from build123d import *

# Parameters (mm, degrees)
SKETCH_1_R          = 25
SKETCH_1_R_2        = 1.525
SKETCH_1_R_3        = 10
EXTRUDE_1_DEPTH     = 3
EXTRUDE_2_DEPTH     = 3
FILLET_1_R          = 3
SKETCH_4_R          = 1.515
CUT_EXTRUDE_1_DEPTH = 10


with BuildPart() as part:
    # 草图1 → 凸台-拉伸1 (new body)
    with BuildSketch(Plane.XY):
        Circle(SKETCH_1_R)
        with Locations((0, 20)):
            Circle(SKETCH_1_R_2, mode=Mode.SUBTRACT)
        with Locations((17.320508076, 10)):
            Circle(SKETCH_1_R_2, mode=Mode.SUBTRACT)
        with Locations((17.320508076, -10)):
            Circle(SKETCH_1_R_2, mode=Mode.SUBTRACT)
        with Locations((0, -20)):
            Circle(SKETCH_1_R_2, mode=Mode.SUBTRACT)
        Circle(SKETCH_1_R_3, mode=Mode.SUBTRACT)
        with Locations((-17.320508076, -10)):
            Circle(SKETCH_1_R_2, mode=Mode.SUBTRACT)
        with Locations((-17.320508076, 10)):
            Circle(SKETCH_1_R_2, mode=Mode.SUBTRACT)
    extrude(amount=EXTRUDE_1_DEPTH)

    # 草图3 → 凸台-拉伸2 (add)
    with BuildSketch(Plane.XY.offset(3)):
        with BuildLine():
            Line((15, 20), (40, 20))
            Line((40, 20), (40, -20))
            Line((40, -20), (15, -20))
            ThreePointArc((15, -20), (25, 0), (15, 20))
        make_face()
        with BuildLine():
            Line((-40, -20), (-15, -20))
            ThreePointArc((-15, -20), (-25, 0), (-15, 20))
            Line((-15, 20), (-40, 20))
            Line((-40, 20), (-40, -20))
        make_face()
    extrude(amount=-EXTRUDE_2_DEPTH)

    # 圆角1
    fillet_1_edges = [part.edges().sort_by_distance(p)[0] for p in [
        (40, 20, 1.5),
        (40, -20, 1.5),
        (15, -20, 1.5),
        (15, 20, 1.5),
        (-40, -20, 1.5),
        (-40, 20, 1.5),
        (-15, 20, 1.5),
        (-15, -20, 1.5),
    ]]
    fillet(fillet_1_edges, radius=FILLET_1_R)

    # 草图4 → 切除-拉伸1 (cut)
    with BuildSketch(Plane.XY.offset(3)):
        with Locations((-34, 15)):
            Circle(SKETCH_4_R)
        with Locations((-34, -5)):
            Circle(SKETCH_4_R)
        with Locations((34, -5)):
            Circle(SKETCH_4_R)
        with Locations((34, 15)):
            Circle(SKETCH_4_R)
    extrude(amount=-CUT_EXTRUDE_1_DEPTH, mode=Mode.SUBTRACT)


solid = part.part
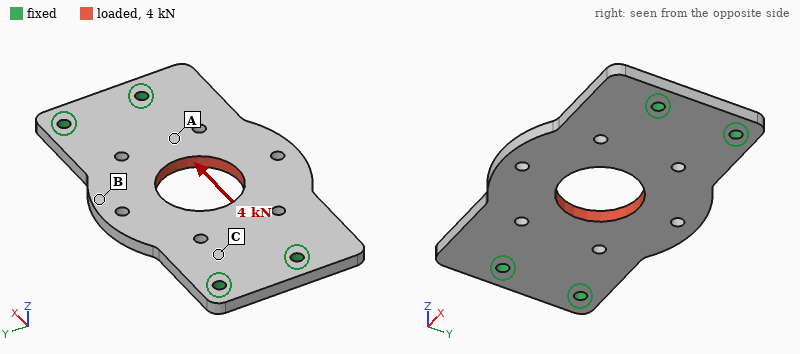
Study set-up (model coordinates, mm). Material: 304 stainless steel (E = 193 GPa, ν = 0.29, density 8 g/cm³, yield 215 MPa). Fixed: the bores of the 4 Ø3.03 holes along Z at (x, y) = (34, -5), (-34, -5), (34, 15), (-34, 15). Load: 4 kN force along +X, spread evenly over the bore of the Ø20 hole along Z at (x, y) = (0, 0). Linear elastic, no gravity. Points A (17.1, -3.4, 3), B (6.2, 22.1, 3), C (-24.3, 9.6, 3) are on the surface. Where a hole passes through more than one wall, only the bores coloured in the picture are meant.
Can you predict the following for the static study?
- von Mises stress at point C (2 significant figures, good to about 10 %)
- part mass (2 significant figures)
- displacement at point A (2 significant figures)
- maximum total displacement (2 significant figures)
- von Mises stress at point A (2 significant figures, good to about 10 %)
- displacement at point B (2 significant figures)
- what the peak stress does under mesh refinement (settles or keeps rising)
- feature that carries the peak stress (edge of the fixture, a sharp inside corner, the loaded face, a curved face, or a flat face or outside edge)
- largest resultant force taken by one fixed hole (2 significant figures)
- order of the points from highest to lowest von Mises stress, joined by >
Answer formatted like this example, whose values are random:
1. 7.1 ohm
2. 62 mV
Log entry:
1. 16 MPa
2. 72 g
3. 2.6 µm
4. 4.7 µm
5. 25 MPa
6. 2.1 µm
7. keeps rising
8. edge of the fixture
9. 1.2 kN
10. A > C > B
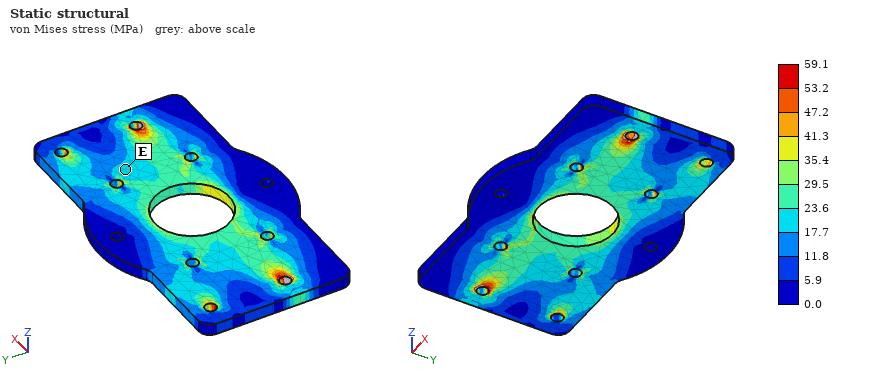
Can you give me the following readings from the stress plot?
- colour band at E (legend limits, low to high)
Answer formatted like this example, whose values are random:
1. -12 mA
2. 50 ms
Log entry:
1. 17.7 to 23.6 MPa
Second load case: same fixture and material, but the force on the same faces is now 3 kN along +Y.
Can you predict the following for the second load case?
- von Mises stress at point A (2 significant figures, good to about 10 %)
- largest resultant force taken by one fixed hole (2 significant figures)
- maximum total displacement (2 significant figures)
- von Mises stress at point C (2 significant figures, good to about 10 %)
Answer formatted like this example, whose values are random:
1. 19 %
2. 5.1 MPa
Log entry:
1. 30 MPa
2. 980 N
3. 8.3 µm
4. 34 MPa
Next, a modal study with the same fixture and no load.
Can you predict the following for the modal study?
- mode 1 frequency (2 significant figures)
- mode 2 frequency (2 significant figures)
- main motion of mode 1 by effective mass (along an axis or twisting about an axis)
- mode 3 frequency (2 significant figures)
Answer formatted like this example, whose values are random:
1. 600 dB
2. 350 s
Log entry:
1. 2900 Hz
2. 3700 Hz
3. along Z
4. 7300 Hz
